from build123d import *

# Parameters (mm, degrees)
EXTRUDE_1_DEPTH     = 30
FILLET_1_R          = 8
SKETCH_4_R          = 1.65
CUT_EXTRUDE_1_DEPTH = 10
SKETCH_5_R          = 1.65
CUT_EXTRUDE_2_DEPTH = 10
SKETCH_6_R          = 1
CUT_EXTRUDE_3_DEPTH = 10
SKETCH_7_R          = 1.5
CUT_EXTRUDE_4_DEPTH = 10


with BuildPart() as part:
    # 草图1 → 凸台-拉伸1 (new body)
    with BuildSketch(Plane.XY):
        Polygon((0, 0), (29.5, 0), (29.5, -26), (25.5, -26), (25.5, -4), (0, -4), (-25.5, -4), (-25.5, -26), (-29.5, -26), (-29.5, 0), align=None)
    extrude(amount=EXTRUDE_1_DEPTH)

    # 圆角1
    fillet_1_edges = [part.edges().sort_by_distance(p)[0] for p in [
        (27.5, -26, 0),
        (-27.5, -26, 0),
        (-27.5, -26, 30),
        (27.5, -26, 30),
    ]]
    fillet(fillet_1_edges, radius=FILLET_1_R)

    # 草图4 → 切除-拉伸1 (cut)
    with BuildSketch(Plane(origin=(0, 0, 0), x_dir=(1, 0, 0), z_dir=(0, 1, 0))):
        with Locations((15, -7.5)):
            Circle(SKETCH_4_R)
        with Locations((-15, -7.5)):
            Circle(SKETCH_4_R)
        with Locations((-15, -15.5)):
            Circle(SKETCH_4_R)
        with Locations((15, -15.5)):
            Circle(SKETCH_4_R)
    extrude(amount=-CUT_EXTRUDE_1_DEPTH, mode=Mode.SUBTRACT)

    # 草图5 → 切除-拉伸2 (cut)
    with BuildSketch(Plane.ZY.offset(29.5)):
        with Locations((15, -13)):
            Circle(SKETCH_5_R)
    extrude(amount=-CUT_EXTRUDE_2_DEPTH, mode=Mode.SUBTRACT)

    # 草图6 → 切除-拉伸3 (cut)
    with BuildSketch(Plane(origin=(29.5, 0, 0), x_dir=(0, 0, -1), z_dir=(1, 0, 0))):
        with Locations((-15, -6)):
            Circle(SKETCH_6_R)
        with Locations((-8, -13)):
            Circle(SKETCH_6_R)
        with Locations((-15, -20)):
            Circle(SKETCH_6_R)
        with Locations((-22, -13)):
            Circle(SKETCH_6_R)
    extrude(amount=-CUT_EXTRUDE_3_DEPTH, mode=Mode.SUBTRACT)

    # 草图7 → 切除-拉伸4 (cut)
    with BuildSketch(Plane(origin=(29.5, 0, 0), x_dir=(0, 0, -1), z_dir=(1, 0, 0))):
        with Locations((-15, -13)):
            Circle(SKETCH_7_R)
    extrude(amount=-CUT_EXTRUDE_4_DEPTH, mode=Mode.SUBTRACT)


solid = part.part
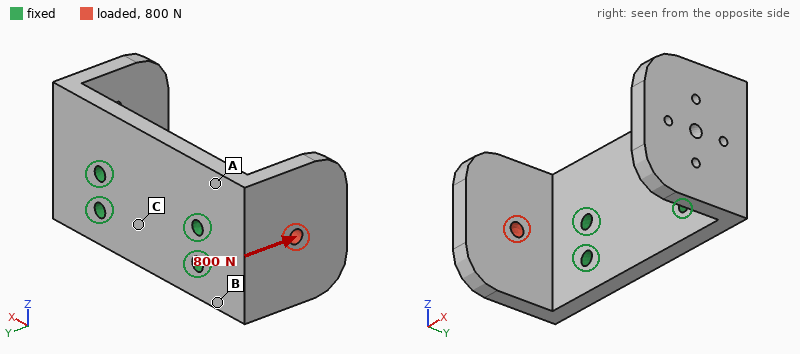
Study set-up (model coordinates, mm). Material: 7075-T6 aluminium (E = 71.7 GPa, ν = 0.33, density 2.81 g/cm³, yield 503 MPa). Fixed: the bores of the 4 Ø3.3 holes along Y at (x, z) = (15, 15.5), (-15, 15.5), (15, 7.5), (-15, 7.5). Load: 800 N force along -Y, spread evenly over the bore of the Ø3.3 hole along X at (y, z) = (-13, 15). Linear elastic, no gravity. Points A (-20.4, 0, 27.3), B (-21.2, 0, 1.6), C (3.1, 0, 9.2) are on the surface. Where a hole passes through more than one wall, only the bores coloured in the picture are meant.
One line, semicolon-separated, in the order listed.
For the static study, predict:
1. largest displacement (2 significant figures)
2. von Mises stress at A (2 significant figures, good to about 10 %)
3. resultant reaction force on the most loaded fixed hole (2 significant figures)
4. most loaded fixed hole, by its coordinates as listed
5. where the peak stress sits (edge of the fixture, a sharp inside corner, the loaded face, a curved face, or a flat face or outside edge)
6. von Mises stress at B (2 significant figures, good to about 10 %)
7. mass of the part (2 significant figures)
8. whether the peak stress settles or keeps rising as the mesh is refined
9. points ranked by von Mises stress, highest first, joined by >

0.15 mm; 44 MPa; 640 N; (-15, 15.5); edge of the fixture; 59 MPa; 33 g; keeps rising; B > A > C
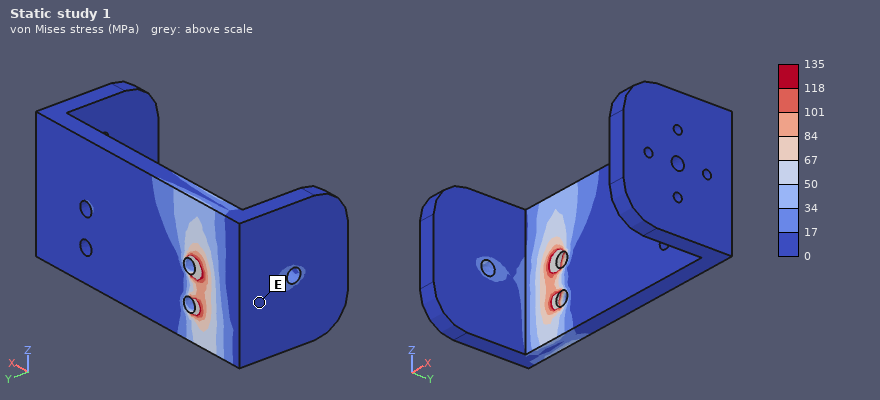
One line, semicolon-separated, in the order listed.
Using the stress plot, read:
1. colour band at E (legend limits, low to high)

0 to 17 MPa
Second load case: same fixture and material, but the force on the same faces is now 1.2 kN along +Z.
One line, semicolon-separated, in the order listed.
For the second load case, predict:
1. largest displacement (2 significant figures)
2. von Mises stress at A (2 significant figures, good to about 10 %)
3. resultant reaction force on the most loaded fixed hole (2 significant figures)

0.16 mm; 32 MPa; 1.3 kN
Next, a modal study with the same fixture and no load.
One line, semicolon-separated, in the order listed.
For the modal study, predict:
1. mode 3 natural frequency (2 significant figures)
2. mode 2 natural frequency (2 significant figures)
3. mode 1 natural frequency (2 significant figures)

5100 Hz; 3300 Hz; 3300 Hz
